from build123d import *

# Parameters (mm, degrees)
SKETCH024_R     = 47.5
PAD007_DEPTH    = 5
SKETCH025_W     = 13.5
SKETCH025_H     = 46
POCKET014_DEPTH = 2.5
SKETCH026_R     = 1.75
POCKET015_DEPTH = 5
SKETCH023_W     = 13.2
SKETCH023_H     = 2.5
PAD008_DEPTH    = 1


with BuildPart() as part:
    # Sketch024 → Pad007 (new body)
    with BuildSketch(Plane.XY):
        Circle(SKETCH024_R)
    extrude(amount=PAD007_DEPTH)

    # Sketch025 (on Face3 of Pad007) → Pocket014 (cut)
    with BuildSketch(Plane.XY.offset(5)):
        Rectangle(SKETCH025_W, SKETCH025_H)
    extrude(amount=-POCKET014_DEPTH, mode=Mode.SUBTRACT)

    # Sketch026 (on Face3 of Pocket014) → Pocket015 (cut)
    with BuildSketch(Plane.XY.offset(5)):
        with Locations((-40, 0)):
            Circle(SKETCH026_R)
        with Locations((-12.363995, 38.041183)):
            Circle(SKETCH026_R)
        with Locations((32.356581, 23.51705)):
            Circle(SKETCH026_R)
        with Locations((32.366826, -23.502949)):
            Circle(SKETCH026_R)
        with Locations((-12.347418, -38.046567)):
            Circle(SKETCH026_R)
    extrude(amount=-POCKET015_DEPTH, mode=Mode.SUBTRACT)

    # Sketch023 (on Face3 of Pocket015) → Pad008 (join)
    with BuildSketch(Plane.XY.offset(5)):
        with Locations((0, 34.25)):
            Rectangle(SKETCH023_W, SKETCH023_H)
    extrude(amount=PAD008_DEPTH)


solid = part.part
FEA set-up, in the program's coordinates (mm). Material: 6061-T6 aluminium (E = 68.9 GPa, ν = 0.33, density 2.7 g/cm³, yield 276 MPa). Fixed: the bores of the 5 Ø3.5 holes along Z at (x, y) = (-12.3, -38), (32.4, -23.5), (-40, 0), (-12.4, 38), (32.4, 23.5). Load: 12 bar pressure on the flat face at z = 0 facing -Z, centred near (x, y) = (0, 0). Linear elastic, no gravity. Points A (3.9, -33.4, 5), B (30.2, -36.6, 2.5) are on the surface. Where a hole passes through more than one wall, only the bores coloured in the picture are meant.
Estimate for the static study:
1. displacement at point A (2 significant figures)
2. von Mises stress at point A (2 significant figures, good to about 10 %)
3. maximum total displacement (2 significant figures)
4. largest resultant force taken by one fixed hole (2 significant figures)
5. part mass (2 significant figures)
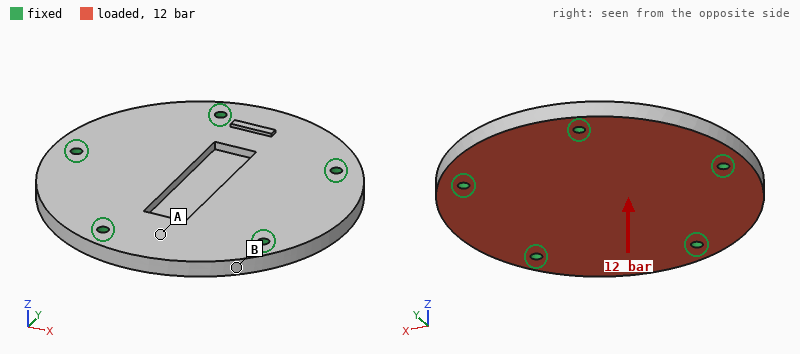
0.039 mm
43 MPa
0.14 mm
1.8 kN
91 g
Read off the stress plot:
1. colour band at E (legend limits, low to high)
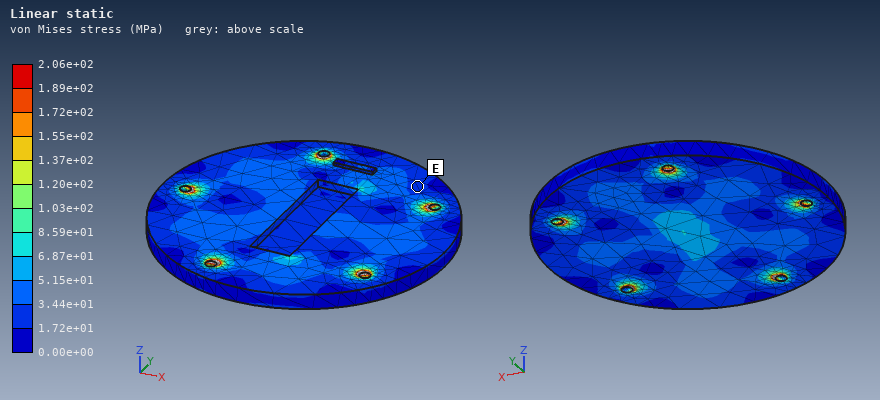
1.72e+01 to 3.44e+01 MPa
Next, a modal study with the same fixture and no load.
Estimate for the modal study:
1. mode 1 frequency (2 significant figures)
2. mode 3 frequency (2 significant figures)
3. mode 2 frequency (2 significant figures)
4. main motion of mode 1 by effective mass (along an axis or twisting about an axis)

5600 Hz
8700 Hz
8700 Hz
along Z
